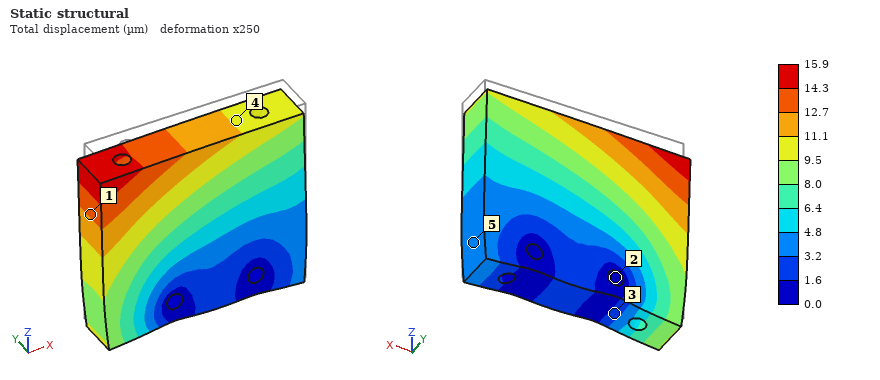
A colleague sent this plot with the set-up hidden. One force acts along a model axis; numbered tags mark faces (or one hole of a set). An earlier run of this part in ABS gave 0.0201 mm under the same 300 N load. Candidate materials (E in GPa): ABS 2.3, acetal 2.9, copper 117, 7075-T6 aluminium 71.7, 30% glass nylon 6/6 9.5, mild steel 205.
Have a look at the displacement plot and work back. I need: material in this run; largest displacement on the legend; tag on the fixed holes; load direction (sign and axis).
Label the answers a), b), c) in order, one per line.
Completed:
a) acetal
b) 15.9 µm
c) 2
d) -Z
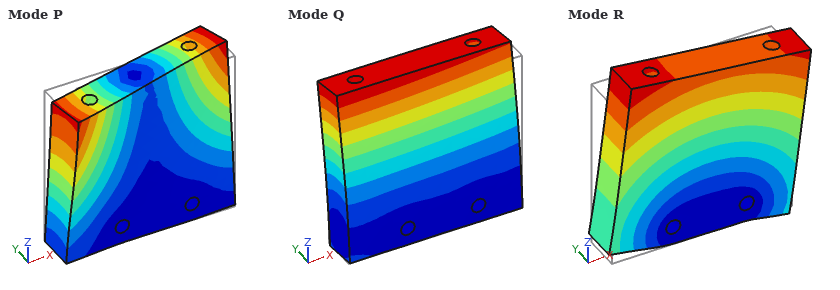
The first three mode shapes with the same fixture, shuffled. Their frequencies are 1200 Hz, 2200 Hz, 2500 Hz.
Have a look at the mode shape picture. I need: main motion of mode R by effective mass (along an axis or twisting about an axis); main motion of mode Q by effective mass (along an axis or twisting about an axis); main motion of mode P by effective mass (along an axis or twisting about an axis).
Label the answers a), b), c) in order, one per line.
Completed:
a) along X
b) along Y
c) twisting about Z
